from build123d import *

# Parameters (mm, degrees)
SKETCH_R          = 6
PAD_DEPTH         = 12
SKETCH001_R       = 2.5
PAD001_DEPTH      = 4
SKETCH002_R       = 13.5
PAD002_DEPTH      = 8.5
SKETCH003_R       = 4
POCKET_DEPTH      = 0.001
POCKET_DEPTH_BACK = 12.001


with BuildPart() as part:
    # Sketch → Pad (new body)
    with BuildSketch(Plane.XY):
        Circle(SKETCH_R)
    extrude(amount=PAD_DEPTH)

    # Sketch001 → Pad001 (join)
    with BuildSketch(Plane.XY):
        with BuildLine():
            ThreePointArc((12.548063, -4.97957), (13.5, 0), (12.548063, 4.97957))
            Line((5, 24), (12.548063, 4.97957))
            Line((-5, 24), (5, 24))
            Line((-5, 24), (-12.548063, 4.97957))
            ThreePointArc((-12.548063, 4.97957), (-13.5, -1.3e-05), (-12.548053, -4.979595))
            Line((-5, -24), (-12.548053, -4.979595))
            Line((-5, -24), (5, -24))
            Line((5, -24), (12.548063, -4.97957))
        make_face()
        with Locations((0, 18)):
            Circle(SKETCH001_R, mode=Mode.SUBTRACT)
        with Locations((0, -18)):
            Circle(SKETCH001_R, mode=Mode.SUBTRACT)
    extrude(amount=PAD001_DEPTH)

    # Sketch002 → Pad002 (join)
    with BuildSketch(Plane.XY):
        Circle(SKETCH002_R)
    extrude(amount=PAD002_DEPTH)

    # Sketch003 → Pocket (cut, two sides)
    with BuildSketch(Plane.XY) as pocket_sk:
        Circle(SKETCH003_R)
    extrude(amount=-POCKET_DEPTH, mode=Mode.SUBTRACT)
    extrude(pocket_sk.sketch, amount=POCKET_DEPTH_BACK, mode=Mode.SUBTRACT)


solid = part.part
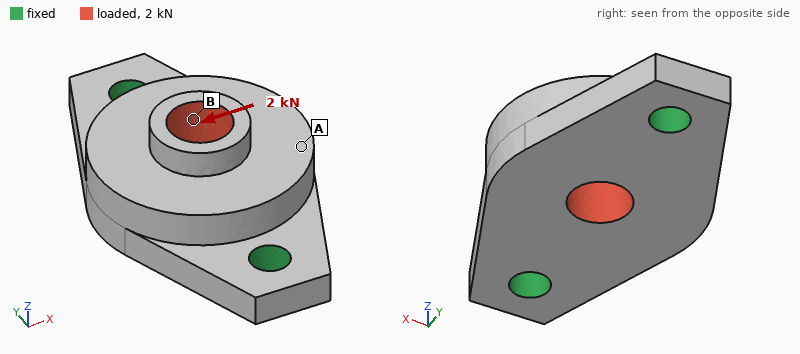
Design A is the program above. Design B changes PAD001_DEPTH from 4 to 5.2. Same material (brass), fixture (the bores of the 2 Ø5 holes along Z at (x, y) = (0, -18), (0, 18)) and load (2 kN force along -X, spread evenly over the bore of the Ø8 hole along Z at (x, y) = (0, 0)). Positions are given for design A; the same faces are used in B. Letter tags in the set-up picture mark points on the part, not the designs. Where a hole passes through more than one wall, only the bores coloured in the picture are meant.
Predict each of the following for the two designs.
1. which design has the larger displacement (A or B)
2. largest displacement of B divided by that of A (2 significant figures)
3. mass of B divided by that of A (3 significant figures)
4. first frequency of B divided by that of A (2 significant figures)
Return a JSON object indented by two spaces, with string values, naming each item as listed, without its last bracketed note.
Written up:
{
  "which design has the larger displacement": "A",
  "largest displacement of B divided by that of A": "0.56",
  "mass of B divided by that of A": "1.06",
  "first frequency of B divided by that of A": "1.3"
}
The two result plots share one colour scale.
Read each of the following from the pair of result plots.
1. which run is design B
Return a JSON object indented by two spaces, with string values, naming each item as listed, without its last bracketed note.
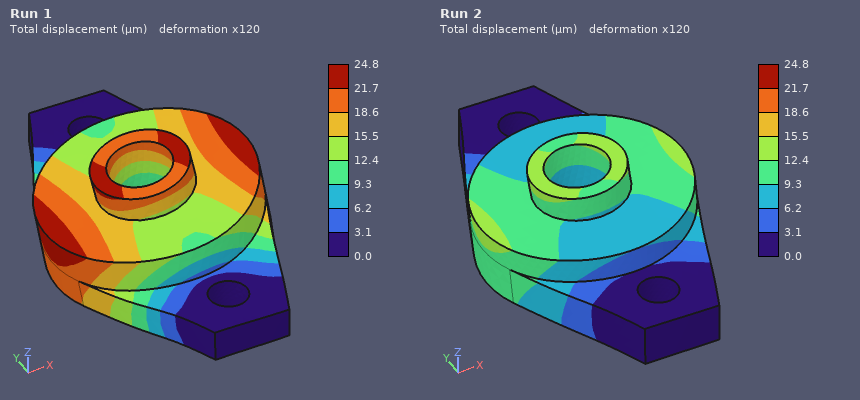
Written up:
{
  "which run is design B": "Run 2"
}
